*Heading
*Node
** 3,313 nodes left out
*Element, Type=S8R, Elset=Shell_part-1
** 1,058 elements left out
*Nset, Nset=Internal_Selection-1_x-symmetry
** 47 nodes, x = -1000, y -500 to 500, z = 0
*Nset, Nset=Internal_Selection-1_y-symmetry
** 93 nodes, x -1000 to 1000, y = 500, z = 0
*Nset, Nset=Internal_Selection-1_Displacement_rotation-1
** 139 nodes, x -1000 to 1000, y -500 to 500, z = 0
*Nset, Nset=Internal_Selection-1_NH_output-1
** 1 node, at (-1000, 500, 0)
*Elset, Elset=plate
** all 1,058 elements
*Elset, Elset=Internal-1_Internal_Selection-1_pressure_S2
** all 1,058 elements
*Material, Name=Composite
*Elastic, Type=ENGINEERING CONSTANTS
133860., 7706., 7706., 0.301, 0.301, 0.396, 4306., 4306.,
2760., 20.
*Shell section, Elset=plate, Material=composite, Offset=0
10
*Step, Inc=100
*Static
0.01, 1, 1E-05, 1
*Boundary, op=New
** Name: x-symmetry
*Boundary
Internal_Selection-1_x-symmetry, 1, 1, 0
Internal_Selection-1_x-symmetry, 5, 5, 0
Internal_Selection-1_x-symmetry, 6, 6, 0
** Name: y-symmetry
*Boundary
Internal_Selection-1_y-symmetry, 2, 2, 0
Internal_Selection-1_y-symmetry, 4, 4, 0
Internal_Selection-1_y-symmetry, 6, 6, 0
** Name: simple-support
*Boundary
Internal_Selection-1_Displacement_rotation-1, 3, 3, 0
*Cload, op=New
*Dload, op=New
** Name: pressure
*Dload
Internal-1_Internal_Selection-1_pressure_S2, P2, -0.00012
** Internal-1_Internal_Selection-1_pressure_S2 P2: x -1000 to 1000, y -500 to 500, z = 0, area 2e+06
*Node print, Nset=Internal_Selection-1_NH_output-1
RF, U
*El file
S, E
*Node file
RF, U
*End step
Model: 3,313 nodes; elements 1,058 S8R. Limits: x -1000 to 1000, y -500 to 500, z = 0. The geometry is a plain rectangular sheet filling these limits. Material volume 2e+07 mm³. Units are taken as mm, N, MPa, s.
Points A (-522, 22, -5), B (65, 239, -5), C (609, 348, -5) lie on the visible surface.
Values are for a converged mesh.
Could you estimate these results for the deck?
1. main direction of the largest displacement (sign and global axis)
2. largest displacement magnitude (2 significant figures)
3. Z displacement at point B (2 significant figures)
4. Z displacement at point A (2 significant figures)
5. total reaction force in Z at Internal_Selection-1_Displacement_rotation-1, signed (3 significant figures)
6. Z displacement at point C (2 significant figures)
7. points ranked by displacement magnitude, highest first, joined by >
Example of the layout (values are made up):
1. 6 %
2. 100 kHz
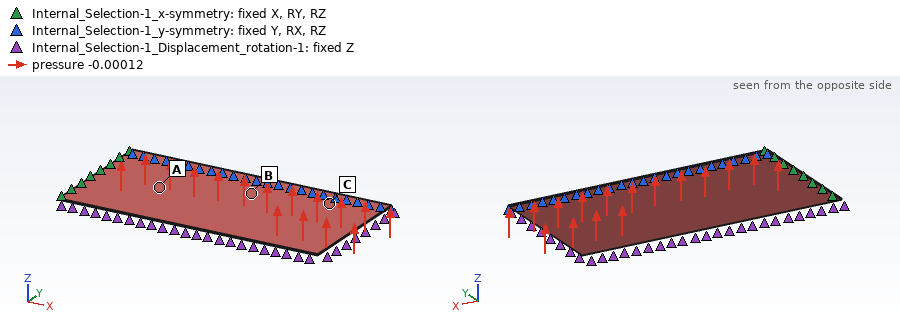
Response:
1. +Z
2. 17 mm
3. 11 mm
4. 12 mm
5. -240 N
6. 5.3 mm
7. A > B > C
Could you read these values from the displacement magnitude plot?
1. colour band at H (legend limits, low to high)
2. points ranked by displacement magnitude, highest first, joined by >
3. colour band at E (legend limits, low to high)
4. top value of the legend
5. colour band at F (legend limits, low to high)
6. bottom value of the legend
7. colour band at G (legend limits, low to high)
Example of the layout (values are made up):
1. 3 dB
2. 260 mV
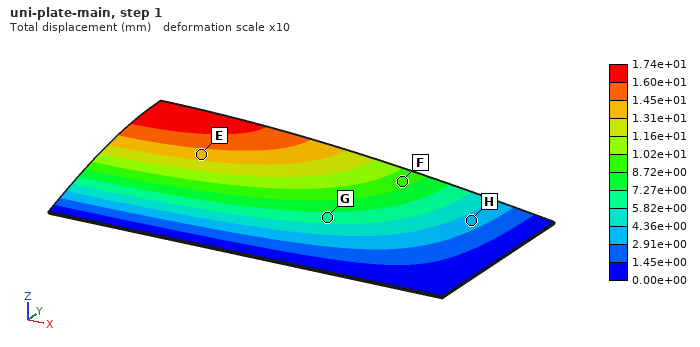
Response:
1. 2.91e+00 to 4.36e+00 mm
2. E > F > G > H
3. 1.31e+01 to 1.45e+01 mm
4. 1.74e+01 mm
5. 8.72e+00 to 1.02e+01 mm
6. 0.00e+00 mm
7. 5.82e+00 to 7.27e+00 mm
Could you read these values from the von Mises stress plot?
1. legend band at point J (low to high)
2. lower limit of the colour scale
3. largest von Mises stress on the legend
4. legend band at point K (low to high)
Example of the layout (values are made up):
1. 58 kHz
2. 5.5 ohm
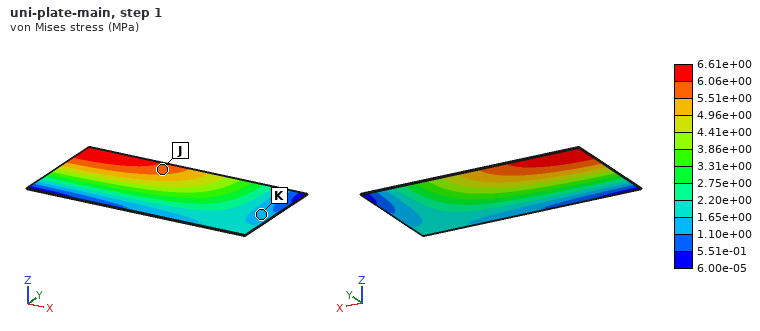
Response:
1. 5.51e+00 to 6.06e+00 MPa
2. 6.00e-05 MPa
3. 6.61e+00 MPa
4. 1.10e+00 to 1.65e+00 MPa
